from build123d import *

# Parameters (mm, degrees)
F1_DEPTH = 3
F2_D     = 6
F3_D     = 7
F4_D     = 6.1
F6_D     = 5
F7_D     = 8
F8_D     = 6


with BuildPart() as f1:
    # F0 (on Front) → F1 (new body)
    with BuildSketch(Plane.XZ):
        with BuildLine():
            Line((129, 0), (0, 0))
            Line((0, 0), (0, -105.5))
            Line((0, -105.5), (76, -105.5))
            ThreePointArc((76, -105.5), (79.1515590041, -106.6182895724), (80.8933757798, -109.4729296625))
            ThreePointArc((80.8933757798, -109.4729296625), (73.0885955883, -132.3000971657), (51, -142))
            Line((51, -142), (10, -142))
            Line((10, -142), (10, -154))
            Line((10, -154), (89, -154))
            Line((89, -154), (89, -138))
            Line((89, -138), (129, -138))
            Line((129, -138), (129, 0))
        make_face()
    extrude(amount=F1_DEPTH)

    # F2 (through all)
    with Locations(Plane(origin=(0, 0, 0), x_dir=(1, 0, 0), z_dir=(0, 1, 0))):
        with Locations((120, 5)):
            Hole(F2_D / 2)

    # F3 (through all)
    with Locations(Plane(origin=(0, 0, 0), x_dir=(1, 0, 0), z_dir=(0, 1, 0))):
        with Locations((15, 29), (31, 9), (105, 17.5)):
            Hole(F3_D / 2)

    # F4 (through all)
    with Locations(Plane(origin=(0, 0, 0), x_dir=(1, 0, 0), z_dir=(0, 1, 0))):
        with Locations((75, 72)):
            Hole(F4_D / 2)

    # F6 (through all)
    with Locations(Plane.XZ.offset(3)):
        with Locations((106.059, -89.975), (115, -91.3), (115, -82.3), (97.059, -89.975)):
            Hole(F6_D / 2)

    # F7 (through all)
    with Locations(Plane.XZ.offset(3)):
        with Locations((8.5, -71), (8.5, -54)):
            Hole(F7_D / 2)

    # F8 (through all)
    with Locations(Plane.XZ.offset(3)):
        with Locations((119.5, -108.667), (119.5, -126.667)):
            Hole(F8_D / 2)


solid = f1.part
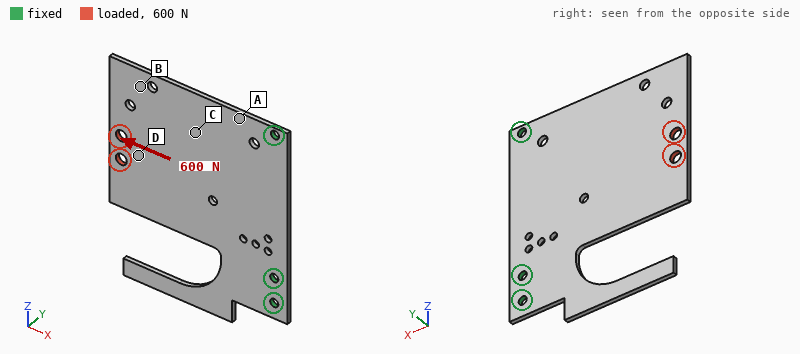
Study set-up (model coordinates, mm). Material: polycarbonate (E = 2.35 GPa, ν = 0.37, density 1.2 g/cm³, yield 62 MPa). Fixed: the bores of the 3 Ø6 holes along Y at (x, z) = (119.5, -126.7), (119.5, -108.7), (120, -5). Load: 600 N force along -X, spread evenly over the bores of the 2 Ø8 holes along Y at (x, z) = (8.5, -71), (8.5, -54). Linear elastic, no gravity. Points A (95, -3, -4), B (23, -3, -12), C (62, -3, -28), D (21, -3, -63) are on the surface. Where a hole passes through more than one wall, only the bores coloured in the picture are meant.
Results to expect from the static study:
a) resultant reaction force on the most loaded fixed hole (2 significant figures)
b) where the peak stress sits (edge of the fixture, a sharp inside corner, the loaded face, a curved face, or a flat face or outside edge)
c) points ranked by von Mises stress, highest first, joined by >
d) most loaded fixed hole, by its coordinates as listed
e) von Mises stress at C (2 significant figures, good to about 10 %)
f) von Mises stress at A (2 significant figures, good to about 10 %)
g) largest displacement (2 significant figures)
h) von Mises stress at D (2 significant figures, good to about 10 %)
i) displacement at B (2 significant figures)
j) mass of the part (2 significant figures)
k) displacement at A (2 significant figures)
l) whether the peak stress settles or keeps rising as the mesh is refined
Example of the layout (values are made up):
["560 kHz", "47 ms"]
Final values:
["300 N", "edge of the fixture", "D > A > C > B", "(120, -5)", "1.9 MPa", "3.3 MPa", "0.21 mm", "4.9 MPa", "0.089 mm", "57 g", "0.050 mm", "keeps rising"]
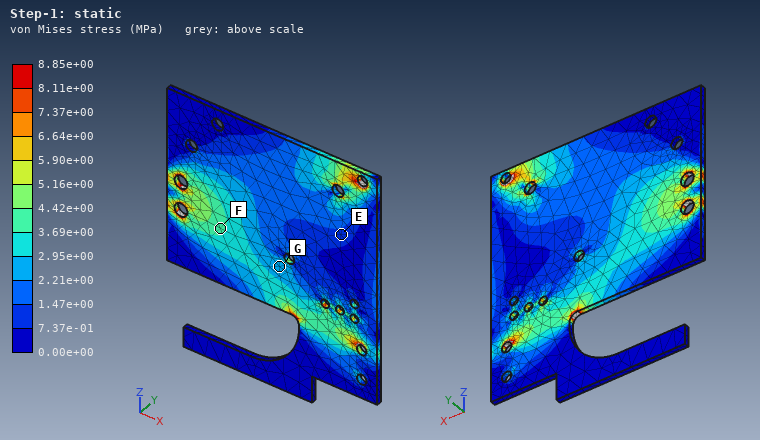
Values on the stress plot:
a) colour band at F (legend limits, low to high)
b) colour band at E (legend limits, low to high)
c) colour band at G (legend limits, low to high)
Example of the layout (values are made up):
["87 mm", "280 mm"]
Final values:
["3.69e+00 to 4.42e+00 MPa", "7.37e-01 to 1.47e+00 MPa", "2.21e+00 to 2.95e+00 MPa"]
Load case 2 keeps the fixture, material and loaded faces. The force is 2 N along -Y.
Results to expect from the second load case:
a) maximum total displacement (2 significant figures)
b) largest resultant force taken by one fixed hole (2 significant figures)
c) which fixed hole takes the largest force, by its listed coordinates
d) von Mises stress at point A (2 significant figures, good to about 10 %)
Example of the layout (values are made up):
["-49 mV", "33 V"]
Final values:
["2.2 mm", "2.1 N", "(119.5, -108.7)", "1.2 MPa"]
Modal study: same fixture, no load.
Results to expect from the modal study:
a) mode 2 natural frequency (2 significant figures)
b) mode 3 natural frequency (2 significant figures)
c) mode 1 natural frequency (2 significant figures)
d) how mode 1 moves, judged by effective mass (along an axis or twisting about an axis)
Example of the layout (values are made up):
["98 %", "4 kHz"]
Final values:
["85 Hz", "140 Hz", "43 Hz", "along Y"]
